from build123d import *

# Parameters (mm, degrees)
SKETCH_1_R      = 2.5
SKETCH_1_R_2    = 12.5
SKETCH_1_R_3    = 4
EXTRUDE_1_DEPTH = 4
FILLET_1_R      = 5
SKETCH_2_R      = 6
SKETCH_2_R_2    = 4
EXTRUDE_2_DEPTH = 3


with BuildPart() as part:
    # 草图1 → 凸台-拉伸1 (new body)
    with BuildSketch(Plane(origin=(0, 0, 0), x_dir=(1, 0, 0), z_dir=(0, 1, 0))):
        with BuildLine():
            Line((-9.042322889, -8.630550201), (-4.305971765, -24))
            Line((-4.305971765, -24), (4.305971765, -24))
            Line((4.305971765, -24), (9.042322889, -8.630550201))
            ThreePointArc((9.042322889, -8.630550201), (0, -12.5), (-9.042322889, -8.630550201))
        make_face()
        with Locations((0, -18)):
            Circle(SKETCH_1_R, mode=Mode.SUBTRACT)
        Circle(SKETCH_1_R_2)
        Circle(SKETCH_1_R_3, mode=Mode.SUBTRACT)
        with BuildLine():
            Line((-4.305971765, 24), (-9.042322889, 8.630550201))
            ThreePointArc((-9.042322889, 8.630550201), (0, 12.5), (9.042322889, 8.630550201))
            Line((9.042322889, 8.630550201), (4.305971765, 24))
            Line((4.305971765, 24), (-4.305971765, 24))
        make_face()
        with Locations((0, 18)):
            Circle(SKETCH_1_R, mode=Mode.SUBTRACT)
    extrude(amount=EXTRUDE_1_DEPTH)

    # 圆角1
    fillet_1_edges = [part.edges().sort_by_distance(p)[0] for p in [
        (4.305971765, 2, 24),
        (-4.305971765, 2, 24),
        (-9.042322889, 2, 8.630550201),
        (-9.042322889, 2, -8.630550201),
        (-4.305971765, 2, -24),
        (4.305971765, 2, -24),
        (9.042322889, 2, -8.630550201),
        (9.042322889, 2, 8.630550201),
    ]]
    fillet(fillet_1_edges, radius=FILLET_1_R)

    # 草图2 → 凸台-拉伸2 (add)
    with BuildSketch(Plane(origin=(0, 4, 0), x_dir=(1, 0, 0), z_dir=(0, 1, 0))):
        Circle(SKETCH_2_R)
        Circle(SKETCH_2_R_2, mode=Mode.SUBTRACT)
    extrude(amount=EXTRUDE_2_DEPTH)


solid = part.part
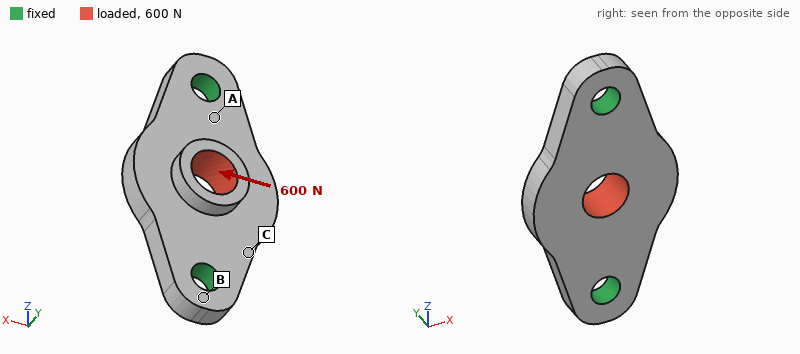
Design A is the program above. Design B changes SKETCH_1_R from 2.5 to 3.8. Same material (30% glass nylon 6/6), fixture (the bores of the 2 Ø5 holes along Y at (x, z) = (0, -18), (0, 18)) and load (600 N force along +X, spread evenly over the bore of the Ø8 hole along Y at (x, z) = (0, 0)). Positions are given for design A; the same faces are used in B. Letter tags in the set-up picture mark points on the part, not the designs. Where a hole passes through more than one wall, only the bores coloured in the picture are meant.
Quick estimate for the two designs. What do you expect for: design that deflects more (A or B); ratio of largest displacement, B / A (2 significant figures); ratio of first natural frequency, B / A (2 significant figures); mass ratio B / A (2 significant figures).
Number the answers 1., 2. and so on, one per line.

1. A
2. 0.78
3. 1.2
4. 0.93
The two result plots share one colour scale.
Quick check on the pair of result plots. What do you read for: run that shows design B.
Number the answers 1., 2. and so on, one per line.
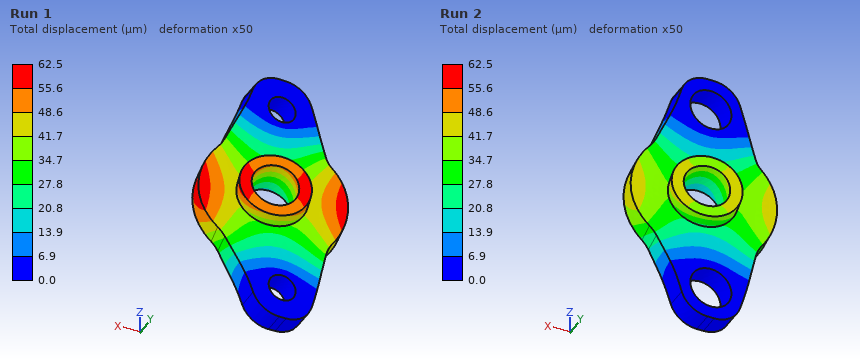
1. Run 2
